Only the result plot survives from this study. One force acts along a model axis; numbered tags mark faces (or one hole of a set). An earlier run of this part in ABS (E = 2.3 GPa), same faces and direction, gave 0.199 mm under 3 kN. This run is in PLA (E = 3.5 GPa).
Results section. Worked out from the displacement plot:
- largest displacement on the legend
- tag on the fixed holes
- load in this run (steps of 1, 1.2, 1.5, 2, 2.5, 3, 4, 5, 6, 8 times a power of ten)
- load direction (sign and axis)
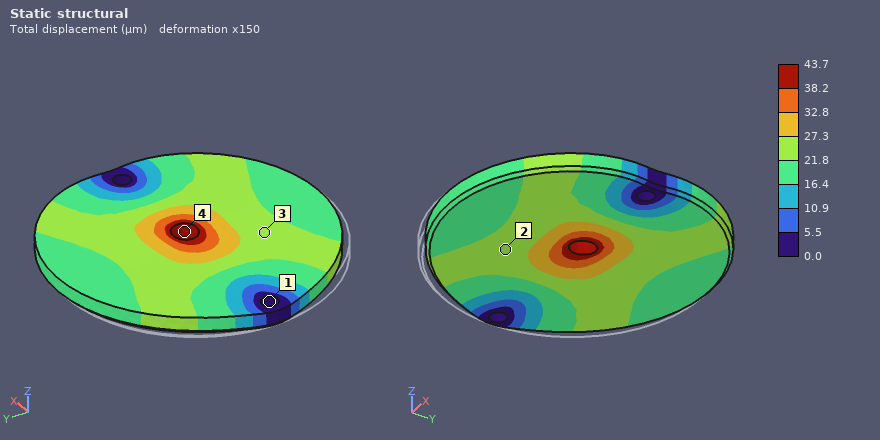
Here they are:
43.7 µm
1
1 kN
+X
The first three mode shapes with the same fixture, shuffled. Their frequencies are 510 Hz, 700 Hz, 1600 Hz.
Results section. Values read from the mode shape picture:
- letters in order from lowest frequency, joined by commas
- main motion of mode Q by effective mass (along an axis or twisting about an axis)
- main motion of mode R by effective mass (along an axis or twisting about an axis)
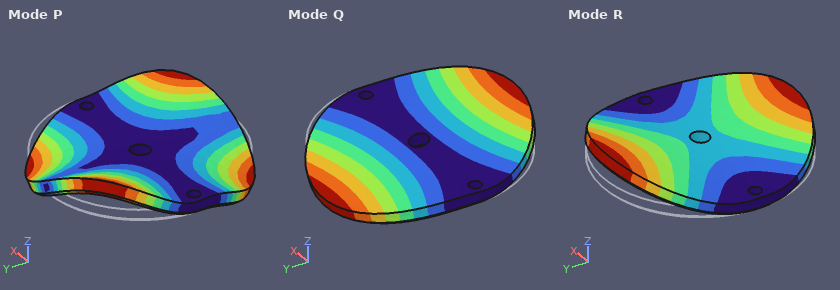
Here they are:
Q, R, P
twisting about X
along Z
